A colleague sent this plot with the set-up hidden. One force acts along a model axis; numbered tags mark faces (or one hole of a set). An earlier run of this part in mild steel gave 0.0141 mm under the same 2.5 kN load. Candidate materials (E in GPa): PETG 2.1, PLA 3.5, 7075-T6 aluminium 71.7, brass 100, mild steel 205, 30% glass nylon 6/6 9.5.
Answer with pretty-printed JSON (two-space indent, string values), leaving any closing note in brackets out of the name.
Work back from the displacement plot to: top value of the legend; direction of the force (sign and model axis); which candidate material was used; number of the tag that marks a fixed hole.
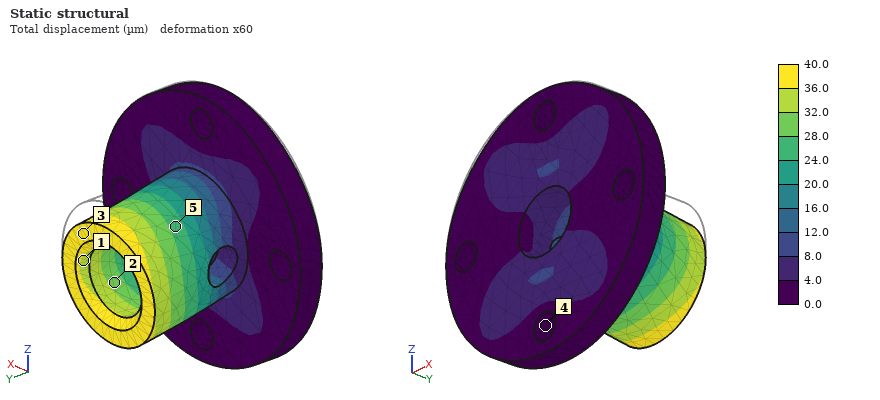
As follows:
{
  "top value of the legend": "40.0 µm",
  "direction of the force": "-Z",
  "which candidate material was used": "7075-T6 aluminium",
  "number of the tag that marks a fixed hole": "4"
}
